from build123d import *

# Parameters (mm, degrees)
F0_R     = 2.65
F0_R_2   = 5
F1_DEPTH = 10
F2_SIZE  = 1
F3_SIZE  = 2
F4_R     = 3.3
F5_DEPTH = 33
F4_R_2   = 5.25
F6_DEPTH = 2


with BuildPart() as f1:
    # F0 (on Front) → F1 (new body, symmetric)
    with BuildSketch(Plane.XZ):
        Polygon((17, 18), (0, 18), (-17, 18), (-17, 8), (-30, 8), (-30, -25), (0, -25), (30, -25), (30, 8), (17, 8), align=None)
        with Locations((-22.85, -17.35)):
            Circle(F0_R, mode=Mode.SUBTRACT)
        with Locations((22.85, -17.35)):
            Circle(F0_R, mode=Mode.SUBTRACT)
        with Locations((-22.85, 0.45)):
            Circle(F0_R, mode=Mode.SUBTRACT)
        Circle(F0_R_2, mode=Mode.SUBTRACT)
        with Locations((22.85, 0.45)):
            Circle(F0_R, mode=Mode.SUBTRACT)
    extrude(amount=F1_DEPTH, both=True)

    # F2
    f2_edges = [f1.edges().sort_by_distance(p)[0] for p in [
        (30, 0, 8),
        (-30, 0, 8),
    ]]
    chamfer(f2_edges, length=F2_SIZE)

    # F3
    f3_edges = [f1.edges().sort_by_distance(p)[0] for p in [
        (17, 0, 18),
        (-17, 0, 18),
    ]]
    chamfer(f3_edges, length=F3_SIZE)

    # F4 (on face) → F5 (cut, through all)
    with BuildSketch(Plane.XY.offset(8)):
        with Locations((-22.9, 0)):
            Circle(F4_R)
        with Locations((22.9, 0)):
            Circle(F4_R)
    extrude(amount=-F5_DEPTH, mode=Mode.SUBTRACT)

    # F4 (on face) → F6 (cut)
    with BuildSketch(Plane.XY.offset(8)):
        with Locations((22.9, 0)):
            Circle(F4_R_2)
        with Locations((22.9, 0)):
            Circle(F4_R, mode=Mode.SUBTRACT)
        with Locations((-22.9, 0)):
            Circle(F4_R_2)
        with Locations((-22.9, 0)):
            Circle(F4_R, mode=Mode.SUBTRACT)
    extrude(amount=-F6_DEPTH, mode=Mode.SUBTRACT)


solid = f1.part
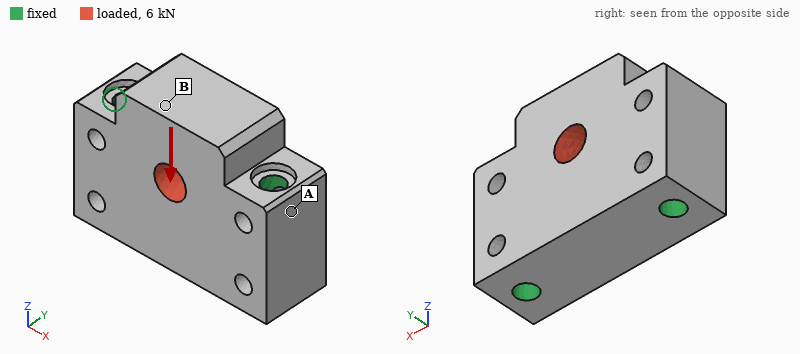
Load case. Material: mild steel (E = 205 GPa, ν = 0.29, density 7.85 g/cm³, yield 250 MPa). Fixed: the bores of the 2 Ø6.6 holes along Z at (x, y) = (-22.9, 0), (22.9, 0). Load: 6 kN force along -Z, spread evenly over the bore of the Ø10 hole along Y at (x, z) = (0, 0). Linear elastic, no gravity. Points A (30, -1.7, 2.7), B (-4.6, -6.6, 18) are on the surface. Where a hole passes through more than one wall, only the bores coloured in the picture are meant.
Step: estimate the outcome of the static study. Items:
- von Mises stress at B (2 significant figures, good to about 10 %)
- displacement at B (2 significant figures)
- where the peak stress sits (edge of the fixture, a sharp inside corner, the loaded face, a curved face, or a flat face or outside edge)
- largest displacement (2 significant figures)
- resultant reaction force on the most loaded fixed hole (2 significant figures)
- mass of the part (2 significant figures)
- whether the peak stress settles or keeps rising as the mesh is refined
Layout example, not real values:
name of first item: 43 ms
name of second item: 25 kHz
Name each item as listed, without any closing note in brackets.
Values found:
von Mises stress at B: 7.5 MPa
displacement at B: 1.2 µm
where the peak stress sits: edge of the fixture
largest displacement: 1.6 µm
resultant reaction force on the most loaded fixed hole: 3.1 kN
mass of the part: 320 g
whether the peak stress settles or keeps rising as the mesh is refined: keeps rising
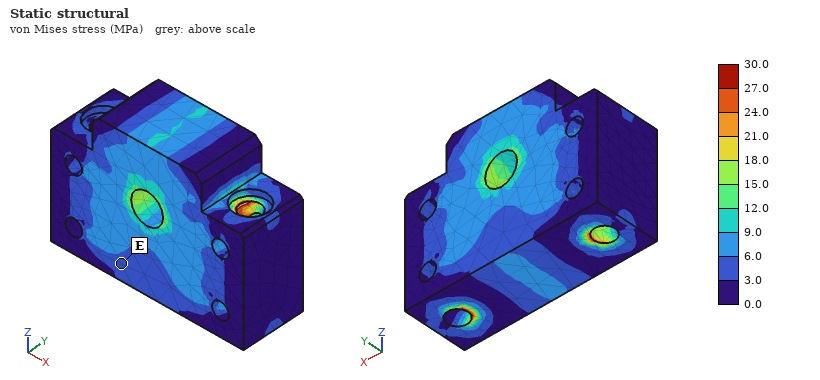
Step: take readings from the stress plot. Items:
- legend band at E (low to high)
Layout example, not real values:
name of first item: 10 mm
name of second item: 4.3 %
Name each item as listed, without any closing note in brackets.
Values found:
legend band at E: 3.0 to 6.0 MPa
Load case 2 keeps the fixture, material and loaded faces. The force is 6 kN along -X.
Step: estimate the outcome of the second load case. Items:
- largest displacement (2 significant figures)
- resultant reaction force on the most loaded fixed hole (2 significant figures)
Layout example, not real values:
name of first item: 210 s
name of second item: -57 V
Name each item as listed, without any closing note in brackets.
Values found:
largest displacement: 1.0 µm
resultant reaction force on the most loaded fixed hole: 3.1 kN
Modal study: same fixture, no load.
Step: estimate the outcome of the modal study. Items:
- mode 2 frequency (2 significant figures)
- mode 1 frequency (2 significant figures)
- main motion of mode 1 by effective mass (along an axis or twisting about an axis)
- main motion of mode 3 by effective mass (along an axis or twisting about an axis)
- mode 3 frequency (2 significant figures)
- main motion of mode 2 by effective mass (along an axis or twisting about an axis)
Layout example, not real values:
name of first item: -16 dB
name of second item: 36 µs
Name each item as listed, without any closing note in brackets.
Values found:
mode 2 frequency: 26 kHz
mode 1 frequency: 17 kHz
main motion of mode 1 by effective mass: along Y
main motion of mode 3 by effective mass: along Z
mode 3 frequency: 29 kHz
main motion of mode 2 by effective mass: along Y
